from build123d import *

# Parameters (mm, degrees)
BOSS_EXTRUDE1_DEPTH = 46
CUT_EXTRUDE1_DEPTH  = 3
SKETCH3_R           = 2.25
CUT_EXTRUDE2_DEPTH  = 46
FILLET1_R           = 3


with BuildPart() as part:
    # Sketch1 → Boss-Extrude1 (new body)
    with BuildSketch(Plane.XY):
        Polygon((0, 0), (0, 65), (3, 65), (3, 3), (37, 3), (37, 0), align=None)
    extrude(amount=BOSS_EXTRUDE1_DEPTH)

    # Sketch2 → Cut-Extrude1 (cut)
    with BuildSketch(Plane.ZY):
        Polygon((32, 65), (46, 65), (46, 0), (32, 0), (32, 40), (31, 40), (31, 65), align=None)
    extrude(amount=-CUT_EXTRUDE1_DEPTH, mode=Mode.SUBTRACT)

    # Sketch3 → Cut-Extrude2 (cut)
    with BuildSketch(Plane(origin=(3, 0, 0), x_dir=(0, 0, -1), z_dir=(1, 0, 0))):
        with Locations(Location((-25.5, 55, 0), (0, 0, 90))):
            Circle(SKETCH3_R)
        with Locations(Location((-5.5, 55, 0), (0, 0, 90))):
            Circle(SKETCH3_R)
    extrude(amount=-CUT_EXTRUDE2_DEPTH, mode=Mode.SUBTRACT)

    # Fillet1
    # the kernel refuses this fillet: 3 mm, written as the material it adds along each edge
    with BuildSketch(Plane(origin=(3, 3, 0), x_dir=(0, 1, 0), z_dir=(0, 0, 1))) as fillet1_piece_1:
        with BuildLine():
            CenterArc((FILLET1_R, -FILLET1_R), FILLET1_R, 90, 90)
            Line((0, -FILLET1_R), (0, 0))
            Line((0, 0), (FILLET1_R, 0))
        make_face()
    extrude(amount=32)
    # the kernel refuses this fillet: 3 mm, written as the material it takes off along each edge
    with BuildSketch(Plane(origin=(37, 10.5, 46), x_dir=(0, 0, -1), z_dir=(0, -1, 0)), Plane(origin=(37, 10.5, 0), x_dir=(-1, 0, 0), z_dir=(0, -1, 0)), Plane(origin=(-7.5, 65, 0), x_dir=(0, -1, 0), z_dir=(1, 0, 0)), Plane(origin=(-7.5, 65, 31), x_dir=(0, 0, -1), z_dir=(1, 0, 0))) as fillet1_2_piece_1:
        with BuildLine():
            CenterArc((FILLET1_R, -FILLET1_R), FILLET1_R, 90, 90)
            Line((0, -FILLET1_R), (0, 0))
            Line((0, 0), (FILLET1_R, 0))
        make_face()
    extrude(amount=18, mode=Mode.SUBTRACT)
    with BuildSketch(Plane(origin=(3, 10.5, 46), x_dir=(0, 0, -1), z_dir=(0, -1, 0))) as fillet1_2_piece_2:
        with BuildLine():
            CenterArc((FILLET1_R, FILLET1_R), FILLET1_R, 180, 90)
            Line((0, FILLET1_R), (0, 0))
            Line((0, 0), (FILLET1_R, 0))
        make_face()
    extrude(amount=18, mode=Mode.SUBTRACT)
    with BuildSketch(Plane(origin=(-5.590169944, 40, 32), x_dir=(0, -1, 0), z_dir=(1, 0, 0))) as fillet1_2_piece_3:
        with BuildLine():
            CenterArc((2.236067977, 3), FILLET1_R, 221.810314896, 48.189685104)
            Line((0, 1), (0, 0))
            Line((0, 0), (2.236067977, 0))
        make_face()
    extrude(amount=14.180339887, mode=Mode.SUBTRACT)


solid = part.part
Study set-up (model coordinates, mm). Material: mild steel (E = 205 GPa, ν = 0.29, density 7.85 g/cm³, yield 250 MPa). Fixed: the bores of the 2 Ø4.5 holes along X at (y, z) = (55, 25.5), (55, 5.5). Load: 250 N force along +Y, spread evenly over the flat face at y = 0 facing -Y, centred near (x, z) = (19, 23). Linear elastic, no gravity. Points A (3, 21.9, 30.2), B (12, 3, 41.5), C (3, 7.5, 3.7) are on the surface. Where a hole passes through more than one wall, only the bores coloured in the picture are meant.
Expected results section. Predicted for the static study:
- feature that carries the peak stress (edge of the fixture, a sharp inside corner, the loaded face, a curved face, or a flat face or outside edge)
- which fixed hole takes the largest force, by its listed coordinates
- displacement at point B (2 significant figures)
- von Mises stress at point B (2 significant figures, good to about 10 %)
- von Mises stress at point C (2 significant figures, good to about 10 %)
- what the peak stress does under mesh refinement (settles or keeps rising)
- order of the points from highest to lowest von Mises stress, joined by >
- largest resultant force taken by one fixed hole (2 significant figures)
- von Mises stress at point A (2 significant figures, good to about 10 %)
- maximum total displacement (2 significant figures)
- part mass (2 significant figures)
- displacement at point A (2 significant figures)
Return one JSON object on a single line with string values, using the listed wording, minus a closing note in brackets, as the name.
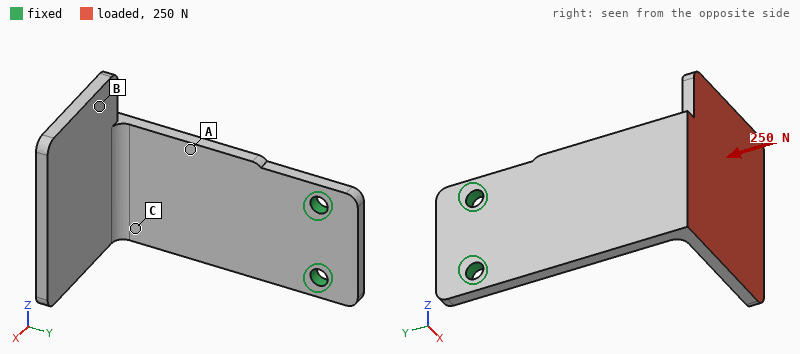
{"feature that carries the peak stress": "edge of the fixture", "which fixed hole takes the largest force, by its listed coordinates": "(55, 25.5)", "displacement at point B": "0.43 mm", "von Mises stress at point B": "12 MPa", "von Mises stress at point C": "76 MPa", "what the peak stress does under mesh refinement": "keeps rising", "order of the points from highest to lowest von Mises stress, joined by >": "A > C > B", "largest resultant force taken by one fixed hole": "210 N", "von Mises stress at point A": "98 MPa", "maximum total displacement": "0.75 mm", "part mass": "85 g", "displacement at point A": "0.15 mm"}
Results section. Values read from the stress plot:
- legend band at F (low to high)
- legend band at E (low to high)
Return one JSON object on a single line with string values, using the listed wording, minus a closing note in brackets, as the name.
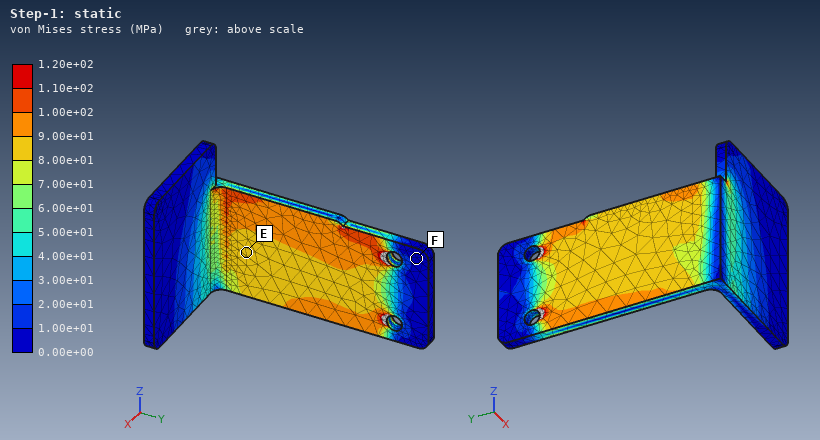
{"legend band at F": "0.00e+00 to 1.00e+01 MPa", "legend band at E": "8.00e+01 to 9.00e+01 MPa"}
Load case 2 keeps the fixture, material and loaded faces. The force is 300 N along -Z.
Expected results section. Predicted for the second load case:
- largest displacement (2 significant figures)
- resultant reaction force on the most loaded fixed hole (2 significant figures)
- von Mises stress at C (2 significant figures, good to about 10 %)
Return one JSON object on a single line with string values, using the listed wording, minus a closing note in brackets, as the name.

{"largest displacement": "0.44 mm", "resultant reaction force on the most loaded fixed hole": "800 N", "von Mises stress at C": "83 MPa"}
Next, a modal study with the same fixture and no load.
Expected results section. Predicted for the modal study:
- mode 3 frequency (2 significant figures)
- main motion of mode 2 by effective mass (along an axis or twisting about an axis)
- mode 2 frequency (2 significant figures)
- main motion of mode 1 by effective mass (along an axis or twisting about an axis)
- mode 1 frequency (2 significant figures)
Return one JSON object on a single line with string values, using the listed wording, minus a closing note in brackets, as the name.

{"mode 3 frequency": "1300 Hz", "main motion of mode 2 by effective mass": "along Z", "mode 2 frequency": "750 Hz", "main motion of mode 1 by effective mass": "along X", "mode 1 frequency": "350 Hz"}
